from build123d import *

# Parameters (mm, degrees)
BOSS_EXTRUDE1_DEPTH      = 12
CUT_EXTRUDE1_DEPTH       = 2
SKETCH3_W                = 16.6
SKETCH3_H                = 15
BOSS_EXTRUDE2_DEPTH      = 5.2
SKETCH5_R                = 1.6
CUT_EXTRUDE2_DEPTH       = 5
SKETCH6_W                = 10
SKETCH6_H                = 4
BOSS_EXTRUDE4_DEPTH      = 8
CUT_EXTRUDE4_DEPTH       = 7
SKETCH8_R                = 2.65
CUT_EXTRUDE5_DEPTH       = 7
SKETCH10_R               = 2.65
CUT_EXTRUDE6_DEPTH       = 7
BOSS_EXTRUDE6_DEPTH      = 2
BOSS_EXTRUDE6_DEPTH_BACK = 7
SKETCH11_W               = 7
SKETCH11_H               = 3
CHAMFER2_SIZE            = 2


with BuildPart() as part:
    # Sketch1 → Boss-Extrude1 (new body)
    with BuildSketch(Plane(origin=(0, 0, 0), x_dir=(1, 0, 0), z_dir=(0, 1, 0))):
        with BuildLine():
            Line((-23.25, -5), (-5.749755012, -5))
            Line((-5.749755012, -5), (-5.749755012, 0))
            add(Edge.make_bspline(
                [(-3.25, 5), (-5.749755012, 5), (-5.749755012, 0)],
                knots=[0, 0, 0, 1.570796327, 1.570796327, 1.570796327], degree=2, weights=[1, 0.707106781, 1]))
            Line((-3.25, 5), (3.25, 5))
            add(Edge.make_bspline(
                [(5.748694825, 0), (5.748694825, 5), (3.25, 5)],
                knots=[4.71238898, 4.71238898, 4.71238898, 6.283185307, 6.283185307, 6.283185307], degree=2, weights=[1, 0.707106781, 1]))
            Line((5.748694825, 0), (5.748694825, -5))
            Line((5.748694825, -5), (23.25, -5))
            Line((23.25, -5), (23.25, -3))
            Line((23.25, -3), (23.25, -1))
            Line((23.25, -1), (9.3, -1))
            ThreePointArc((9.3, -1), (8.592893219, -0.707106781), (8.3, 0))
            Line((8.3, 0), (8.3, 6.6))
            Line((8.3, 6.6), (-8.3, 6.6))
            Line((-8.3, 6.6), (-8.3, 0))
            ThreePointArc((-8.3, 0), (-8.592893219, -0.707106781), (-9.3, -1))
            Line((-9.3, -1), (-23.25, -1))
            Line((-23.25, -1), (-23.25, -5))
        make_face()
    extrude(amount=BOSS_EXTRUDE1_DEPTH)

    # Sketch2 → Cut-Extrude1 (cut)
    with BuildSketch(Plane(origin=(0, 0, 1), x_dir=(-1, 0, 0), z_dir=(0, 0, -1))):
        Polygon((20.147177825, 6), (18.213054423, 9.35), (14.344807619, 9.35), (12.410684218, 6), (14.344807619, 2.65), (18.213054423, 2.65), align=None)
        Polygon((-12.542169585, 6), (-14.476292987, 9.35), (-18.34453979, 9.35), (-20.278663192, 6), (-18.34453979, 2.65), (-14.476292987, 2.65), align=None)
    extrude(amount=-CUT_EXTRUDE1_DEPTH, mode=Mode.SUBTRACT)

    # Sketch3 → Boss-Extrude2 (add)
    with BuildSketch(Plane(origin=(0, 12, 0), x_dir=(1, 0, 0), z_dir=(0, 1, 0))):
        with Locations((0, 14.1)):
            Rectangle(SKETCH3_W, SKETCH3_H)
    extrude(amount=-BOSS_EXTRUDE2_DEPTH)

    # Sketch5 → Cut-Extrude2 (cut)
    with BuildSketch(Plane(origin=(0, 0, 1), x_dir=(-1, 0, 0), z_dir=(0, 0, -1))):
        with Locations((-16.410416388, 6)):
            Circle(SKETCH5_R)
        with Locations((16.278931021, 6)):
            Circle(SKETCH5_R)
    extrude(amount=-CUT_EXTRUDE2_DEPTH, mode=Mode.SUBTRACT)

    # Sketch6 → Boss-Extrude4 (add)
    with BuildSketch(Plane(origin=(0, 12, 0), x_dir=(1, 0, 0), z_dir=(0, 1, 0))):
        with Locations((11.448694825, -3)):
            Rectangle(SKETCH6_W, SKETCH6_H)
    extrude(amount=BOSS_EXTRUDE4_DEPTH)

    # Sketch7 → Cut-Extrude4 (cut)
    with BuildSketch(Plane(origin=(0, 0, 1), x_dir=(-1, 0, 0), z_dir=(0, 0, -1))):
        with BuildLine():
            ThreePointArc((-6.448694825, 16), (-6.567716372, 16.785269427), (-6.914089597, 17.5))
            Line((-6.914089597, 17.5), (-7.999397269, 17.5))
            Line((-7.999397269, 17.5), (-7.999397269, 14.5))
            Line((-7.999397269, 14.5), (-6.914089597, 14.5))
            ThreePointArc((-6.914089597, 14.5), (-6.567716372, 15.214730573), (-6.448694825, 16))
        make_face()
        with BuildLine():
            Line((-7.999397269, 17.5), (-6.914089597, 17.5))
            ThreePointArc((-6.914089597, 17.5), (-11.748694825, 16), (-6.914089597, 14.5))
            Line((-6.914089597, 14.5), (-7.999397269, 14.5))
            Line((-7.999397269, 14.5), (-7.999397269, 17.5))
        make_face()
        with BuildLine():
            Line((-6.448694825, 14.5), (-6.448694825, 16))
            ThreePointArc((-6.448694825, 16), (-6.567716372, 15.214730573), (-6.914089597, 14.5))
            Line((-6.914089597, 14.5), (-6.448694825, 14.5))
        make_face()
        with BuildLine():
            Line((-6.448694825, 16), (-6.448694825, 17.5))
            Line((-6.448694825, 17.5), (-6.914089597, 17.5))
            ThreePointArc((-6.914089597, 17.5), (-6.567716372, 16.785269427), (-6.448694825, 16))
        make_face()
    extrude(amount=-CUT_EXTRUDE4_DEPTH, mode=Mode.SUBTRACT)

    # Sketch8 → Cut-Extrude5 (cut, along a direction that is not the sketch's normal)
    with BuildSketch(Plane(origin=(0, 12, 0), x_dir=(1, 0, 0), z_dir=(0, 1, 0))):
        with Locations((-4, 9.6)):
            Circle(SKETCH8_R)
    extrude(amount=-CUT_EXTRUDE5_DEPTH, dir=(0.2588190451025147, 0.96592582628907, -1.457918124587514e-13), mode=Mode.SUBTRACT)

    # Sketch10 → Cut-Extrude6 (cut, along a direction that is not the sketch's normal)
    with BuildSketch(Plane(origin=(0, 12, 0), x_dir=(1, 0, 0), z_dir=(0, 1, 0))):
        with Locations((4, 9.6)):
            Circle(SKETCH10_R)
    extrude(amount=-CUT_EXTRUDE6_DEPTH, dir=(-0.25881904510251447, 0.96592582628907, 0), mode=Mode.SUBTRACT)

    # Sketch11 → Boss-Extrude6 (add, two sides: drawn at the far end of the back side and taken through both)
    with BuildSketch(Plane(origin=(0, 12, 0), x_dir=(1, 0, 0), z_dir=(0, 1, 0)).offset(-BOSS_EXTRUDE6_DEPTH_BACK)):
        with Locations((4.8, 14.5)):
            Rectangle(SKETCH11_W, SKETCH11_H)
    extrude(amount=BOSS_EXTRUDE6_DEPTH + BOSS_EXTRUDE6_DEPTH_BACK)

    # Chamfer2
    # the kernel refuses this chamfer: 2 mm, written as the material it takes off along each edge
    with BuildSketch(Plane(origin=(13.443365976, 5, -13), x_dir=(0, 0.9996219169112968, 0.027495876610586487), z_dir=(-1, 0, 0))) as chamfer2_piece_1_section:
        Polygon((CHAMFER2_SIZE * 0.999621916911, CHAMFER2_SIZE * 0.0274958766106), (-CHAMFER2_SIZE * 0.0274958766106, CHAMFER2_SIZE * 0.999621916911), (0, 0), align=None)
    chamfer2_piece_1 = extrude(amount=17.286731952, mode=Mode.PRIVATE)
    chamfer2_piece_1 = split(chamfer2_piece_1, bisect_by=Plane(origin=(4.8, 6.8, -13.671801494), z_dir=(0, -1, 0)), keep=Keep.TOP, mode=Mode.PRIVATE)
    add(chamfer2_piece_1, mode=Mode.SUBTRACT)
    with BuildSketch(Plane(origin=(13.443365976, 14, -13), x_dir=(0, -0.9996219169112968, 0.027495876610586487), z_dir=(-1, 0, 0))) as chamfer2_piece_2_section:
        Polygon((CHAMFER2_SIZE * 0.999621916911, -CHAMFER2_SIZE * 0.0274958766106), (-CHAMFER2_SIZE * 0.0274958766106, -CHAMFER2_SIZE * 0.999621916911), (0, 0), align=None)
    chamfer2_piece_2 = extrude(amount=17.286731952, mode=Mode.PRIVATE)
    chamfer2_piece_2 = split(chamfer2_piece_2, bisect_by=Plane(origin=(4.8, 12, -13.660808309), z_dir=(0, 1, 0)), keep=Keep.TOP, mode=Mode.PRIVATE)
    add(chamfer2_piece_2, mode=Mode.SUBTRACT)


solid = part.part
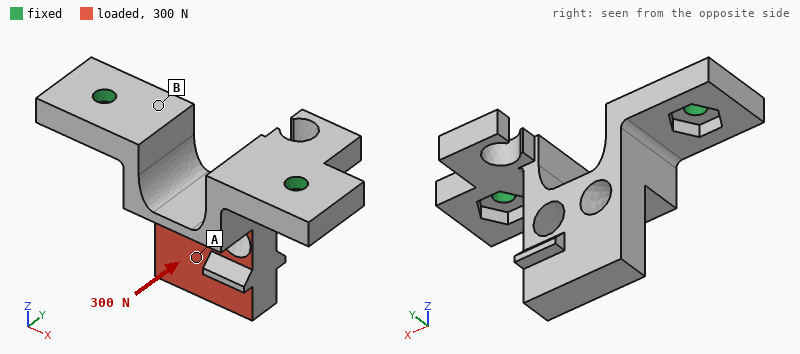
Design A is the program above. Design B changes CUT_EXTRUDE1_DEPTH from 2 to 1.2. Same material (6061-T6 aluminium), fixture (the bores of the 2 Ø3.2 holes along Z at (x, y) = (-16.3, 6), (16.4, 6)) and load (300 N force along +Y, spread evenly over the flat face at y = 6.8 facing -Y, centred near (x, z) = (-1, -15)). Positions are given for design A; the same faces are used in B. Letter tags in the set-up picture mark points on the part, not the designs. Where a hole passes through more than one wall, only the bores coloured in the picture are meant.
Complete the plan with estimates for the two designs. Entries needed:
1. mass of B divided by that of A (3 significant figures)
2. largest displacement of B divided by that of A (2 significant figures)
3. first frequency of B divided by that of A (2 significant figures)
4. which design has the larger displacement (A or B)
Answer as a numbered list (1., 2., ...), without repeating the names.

1. 1.01
2. 0.78
3. 1.2
4. A
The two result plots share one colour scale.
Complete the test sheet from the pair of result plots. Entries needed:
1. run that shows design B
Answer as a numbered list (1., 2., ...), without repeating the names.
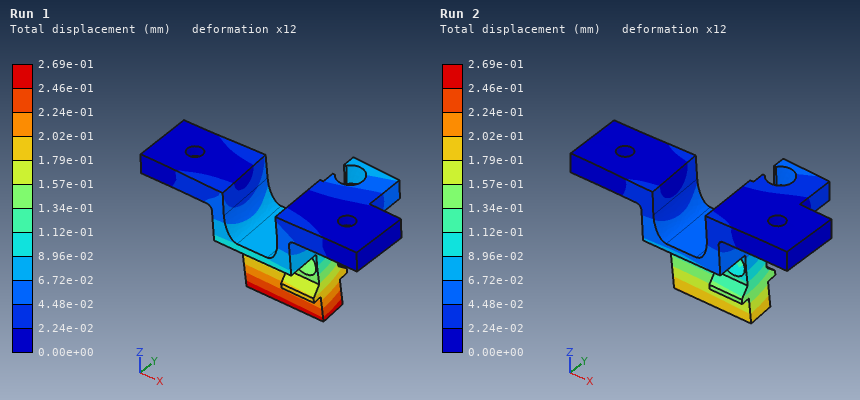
1. Run 2
